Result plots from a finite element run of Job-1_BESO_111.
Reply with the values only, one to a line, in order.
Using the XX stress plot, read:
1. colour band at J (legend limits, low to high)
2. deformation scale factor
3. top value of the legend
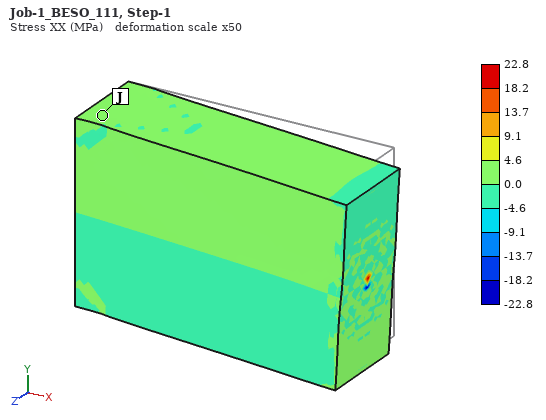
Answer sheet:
0.0 to 4.6 MPa
50
22.8 MPa
